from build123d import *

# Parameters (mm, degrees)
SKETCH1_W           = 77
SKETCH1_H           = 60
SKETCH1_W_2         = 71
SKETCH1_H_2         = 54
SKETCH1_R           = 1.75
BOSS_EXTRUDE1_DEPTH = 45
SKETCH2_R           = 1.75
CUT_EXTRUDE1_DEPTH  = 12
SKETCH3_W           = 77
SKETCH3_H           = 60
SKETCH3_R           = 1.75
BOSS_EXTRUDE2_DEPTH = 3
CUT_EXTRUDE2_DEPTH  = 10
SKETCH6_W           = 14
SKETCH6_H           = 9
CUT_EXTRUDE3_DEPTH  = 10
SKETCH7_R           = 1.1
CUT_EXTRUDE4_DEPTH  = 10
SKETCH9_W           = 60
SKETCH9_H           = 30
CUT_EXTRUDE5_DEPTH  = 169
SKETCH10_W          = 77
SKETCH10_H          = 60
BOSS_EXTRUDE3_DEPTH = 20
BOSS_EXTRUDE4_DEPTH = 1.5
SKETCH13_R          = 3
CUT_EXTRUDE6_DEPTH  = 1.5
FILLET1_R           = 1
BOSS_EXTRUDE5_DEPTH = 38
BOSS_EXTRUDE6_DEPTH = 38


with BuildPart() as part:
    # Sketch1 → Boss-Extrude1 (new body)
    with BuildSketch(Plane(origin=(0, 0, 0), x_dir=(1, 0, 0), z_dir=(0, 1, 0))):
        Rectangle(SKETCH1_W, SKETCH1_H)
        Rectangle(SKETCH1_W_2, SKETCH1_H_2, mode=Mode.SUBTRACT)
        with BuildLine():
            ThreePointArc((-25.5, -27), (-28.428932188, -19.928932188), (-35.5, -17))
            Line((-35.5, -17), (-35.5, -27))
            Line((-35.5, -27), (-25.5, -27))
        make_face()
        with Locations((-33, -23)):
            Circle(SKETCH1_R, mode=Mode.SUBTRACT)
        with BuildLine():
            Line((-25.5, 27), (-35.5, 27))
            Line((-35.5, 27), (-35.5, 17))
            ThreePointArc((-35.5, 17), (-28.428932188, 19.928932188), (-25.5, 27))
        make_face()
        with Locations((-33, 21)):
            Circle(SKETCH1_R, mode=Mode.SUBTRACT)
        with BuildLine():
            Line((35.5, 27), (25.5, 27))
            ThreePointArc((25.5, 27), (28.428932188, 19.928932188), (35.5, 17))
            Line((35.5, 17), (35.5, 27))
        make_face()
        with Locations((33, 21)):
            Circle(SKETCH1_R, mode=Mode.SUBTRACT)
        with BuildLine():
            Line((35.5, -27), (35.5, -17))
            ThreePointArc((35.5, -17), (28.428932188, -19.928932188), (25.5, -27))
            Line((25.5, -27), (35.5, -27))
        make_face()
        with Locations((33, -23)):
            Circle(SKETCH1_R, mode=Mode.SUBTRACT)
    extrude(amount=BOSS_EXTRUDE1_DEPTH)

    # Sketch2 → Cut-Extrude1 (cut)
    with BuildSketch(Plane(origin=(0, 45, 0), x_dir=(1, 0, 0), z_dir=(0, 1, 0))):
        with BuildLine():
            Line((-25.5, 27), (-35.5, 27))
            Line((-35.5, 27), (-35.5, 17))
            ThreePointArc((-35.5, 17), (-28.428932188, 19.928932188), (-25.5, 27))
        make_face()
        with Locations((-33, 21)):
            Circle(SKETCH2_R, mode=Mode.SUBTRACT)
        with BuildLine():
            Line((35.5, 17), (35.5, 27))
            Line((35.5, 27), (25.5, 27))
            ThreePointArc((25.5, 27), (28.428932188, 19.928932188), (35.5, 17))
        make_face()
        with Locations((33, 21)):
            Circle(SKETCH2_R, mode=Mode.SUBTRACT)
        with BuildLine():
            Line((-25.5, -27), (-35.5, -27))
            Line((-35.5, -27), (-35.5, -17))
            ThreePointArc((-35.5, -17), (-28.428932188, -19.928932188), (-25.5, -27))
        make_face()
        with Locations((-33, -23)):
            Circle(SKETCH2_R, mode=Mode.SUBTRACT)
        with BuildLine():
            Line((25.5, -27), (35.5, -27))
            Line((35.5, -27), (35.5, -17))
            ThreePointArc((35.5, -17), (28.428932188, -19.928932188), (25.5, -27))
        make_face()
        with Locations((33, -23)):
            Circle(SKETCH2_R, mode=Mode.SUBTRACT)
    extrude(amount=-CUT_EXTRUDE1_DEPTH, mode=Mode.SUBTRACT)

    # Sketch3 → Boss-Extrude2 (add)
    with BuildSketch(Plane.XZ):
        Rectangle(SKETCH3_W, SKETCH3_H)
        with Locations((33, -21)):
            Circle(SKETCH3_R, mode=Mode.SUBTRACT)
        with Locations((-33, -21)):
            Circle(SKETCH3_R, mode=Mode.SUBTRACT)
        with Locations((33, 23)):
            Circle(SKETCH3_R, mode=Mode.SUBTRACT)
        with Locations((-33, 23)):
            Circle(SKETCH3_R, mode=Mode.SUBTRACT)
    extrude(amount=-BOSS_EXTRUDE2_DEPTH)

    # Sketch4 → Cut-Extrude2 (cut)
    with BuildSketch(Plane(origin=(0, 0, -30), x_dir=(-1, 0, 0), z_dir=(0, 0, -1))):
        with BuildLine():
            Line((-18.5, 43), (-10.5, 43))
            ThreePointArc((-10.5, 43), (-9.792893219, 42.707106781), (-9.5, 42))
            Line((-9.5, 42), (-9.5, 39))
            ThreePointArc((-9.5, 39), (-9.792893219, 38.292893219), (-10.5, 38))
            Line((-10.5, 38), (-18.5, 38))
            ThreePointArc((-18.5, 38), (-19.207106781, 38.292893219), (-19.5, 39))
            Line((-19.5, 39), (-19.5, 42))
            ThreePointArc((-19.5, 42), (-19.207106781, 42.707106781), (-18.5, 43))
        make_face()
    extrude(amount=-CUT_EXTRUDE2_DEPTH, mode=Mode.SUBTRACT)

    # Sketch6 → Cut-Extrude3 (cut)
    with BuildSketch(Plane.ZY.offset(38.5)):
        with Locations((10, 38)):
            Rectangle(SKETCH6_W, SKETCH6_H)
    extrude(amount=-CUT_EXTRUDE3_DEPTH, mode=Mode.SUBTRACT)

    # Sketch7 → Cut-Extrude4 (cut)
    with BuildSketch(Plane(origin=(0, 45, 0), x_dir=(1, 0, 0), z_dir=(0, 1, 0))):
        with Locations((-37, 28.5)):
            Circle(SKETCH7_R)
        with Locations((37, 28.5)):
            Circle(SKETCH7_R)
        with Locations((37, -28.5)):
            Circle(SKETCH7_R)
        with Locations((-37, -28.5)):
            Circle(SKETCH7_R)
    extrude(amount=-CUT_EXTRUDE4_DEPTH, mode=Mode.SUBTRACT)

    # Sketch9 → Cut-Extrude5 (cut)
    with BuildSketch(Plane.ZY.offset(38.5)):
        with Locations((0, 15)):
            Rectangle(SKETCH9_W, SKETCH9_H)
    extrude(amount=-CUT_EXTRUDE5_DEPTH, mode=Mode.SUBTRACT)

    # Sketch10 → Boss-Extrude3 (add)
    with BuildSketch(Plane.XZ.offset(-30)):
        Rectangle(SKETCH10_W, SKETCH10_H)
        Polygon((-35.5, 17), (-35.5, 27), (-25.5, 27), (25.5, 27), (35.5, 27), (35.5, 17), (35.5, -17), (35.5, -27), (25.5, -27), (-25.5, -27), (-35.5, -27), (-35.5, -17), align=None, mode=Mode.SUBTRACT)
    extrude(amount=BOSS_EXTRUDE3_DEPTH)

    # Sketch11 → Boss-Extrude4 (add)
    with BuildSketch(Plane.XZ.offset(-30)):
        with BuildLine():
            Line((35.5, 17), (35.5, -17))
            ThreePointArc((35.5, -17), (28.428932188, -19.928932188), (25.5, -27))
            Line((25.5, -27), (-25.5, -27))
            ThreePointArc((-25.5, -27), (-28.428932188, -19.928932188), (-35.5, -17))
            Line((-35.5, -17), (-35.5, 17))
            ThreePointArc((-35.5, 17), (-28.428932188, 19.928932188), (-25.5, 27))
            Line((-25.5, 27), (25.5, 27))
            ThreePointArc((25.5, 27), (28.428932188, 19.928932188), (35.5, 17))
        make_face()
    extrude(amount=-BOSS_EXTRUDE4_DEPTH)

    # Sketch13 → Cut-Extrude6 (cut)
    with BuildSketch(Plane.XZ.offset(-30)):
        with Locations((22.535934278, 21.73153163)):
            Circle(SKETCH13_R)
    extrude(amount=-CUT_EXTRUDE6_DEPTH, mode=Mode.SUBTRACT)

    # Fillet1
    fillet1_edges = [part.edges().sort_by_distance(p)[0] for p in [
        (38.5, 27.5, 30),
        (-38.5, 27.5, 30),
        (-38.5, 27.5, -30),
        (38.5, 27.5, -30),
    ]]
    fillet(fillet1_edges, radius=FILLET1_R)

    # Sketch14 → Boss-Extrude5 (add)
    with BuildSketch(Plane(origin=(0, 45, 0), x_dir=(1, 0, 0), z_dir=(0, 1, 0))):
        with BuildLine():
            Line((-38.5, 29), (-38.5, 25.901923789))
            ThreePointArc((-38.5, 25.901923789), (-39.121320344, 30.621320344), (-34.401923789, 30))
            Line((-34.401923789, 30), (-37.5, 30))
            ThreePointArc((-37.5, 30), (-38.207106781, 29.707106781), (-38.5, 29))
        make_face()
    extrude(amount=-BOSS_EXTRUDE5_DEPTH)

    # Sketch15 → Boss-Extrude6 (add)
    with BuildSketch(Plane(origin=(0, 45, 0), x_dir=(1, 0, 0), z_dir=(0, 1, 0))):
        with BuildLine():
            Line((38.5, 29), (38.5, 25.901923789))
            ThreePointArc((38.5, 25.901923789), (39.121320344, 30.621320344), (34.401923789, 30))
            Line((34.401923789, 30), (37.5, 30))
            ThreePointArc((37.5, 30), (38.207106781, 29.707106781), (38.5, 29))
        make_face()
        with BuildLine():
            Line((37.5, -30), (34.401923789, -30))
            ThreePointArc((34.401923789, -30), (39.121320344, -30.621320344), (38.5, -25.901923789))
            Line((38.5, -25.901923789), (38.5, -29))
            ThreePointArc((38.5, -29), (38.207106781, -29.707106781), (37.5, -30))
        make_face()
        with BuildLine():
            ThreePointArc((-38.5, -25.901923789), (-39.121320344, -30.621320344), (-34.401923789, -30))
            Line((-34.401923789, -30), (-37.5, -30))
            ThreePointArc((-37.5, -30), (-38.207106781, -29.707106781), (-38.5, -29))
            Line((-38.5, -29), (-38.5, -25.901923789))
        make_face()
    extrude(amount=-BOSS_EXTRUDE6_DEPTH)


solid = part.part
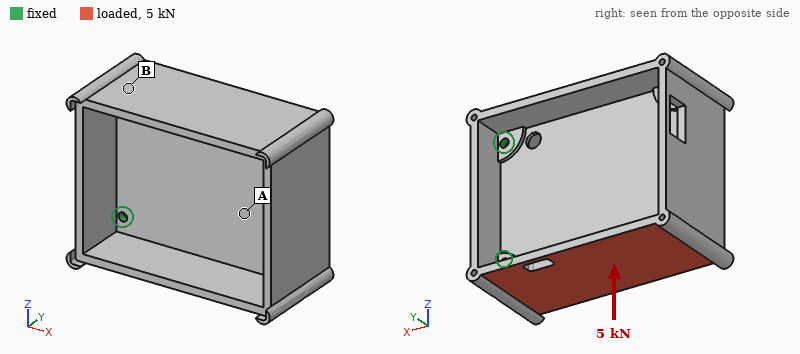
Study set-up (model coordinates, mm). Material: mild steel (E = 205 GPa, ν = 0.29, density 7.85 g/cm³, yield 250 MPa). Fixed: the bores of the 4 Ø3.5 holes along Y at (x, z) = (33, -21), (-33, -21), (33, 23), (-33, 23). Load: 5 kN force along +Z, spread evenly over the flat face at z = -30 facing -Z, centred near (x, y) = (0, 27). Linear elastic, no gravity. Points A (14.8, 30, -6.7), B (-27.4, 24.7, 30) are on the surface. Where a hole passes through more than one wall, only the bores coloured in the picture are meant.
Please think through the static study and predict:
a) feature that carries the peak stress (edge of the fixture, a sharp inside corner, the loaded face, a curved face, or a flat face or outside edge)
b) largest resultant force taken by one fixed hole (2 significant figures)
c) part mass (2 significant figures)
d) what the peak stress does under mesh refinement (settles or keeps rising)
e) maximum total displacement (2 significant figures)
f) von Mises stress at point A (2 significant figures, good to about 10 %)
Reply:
edge of the fixture
1.7 kN
270 g
keeps rising
0.13 mm
35 MPa
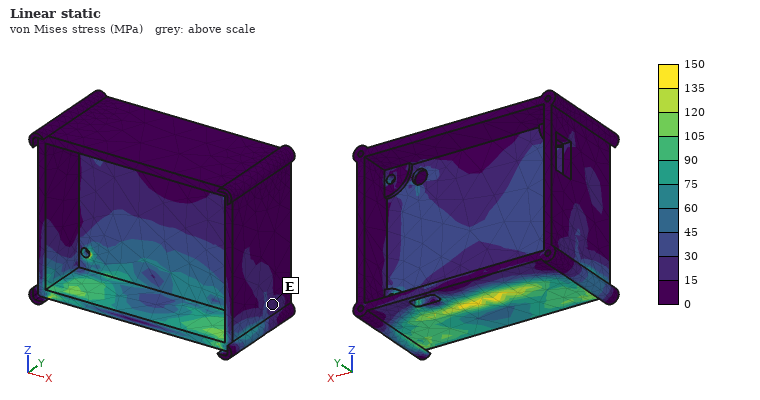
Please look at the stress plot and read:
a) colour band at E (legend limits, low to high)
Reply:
15 to 30 MPa
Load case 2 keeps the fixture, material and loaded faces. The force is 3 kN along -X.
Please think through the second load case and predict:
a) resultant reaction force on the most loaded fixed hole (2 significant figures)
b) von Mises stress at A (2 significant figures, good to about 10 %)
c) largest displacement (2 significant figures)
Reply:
1.5 kN
7.6 MPa
5.3 µm
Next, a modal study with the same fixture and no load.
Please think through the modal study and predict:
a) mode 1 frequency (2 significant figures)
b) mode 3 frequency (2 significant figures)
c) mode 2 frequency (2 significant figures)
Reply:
3300 Hz
4800 Hz
4600 Hz
